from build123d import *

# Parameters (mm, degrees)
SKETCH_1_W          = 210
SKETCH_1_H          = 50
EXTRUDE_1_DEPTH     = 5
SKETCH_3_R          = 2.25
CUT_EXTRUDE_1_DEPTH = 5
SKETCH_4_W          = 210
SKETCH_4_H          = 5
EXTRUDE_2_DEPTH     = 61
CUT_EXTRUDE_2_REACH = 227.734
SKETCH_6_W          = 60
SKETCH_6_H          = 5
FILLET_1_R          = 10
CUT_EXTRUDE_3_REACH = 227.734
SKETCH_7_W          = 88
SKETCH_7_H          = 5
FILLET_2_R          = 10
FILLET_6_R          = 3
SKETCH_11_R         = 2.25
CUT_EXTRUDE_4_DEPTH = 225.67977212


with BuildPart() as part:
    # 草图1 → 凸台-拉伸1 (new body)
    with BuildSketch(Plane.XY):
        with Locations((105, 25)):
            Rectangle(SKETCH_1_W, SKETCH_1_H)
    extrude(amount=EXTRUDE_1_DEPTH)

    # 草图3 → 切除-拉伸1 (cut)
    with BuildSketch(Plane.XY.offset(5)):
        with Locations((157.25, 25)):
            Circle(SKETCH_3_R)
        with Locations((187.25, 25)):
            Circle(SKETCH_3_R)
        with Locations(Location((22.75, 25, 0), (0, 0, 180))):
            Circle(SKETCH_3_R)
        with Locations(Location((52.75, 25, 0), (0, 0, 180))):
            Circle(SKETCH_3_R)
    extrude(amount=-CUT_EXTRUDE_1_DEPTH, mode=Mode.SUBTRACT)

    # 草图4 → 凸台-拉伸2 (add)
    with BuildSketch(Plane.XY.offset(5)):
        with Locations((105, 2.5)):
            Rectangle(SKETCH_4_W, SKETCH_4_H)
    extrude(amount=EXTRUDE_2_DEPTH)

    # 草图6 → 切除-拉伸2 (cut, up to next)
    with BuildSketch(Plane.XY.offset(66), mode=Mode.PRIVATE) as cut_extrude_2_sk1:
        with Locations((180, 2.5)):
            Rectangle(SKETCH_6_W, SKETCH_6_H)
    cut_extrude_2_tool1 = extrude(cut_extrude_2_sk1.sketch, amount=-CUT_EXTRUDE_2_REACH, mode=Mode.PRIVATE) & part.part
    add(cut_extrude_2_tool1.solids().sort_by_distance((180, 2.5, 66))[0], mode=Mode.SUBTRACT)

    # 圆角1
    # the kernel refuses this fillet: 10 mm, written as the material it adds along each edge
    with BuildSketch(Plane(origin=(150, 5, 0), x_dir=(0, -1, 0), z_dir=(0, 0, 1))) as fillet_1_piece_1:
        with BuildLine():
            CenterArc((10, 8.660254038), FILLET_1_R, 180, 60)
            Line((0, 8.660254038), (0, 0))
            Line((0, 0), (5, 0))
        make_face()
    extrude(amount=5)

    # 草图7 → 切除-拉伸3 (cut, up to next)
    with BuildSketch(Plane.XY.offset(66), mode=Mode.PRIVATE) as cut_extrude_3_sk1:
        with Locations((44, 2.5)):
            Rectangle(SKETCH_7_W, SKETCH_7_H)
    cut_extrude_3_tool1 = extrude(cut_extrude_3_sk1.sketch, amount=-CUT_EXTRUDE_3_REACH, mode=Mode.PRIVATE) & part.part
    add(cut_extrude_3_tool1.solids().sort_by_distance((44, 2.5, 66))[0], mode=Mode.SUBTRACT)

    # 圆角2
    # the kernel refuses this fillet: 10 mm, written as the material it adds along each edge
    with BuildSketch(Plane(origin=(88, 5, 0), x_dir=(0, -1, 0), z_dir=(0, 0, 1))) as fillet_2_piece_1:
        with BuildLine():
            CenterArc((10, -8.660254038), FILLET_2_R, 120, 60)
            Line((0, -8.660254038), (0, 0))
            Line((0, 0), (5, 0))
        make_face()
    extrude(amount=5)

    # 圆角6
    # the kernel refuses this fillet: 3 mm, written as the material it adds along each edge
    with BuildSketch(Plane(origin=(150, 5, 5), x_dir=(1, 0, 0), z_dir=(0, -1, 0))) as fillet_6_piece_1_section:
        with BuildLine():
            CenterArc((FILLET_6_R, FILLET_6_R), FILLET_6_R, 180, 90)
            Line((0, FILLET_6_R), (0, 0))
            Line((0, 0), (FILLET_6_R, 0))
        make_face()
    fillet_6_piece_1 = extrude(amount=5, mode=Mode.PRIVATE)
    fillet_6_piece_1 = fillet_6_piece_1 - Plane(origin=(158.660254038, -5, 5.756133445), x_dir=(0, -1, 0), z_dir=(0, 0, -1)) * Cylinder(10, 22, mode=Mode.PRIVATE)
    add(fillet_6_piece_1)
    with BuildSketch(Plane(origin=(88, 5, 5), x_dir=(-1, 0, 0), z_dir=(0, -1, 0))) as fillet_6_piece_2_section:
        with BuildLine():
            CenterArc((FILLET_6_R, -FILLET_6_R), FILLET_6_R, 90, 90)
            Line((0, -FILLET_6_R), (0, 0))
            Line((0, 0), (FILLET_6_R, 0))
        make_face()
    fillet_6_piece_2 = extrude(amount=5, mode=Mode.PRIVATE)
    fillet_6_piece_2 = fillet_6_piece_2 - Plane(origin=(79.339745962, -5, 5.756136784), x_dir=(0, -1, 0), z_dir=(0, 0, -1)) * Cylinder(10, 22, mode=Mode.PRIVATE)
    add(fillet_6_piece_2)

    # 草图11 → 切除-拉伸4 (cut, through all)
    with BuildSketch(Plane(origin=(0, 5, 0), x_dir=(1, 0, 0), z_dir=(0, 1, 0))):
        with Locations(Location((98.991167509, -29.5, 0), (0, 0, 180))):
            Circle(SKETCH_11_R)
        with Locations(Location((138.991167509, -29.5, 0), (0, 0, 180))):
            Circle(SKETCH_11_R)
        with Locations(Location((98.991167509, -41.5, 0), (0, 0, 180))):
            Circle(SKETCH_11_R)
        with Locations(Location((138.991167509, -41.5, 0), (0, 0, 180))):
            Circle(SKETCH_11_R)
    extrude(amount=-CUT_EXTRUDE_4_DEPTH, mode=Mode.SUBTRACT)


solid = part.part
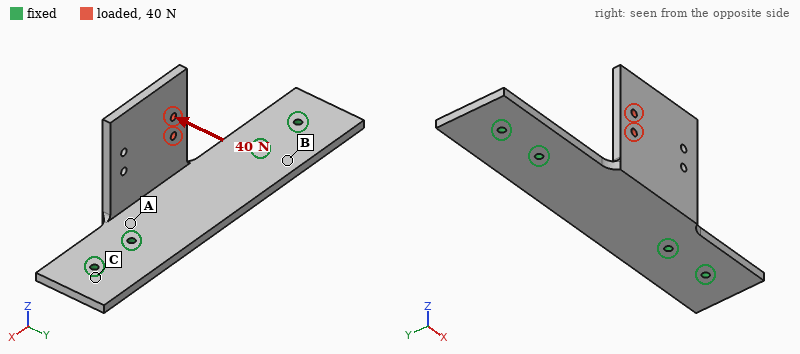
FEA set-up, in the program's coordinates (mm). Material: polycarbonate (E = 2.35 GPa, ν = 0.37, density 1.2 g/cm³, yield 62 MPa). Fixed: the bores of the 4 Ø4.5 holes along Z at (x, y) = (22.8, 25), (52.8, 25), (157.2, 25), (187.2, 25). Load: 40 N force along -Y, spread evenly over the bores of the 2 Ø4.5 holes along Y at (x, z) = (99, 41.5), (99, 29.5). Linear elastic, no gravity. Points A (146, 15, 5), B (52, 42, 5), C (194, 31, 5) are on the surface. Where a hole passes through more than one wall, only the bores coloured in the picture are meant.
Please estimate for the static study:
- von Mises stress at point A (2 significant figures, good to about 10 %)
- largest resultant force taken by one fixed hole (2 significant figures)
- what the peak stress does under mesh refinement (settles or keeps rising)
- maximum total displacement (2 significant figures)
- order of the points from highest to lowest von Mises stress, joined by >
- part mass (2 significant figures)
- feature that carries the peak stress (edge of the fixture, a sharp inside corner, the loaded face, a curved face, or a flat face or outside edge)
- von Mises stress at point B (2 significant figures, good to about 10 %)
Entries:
3.2 MPa
31 N
keeps rising
2.3 mm
A > B > C
81 g
edge of the fixture
1.3 MPa
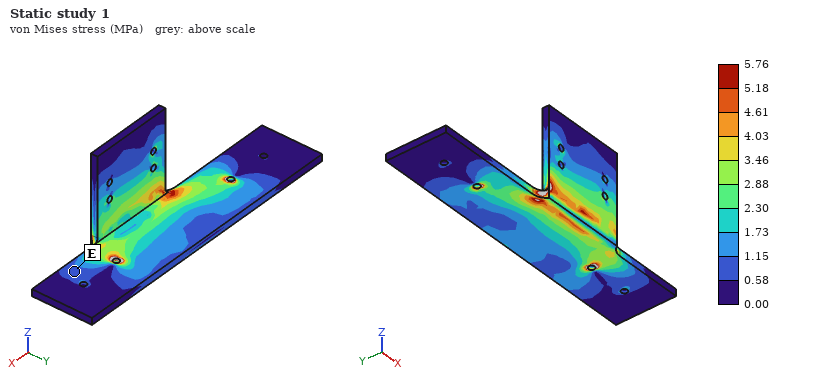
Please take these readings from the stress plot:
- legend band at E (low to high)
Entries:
0.58 to 1.15 MPa
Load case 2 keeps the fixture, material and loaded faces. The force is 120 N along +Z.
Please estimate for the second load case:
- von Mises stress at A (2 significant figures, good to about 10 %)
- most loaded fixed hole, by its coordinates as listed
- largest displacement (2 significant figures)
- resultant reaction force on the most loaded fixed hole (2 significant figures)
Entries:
4.2 MPa
(52.8, 25)
2.4 mm
94 N
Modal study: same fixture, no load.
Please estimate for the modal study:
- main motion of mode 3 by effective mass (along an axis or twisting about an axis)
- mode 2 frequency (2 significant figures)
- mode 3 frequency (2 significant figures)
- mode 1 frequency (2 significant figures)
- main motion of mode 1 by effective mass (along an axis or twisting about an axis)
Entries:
along Z
390 Hz
580 Hz
180 Hz
along Y
